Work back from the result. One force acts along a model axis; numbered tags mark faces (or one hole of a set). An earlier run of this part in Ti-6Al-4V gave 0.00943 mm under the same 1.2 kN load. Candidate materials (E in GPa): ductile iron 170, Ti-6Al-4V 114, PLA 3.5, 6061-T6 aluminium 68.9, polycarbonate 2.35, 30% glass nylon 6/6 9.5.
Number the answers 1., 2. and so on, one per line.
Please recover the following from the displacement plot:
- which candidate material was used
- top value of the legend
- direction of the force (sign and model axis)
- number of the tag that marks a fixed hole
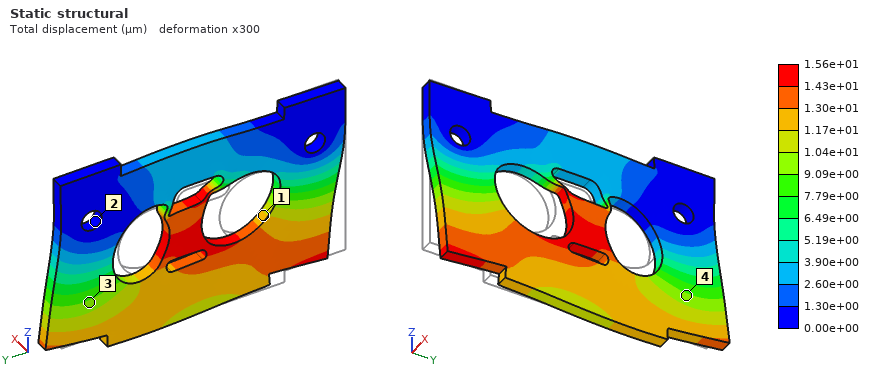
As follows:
1. 6061-T6 aluminium
2. 1.56e+01 µm
3. +Y
4. 2
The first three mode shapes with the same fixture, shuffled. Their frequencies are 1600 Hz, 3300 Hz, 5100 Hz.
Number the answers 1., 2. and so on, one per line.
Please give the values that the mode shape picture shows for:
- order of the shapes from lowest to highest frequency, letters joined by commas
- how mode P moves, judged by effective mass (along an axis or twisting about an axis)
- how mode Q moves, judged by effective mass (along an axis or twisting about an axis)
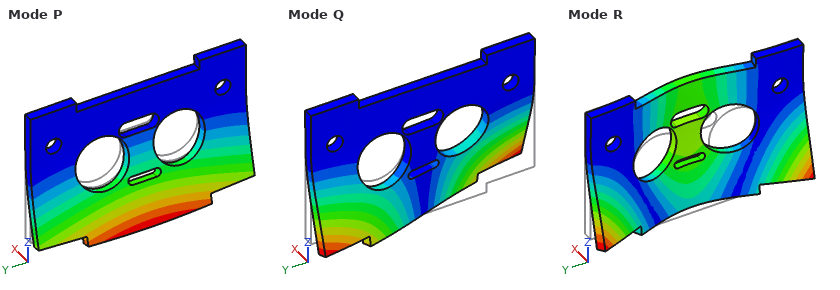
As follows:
1. P, Q, R
2. along X
3. twisting about Z
